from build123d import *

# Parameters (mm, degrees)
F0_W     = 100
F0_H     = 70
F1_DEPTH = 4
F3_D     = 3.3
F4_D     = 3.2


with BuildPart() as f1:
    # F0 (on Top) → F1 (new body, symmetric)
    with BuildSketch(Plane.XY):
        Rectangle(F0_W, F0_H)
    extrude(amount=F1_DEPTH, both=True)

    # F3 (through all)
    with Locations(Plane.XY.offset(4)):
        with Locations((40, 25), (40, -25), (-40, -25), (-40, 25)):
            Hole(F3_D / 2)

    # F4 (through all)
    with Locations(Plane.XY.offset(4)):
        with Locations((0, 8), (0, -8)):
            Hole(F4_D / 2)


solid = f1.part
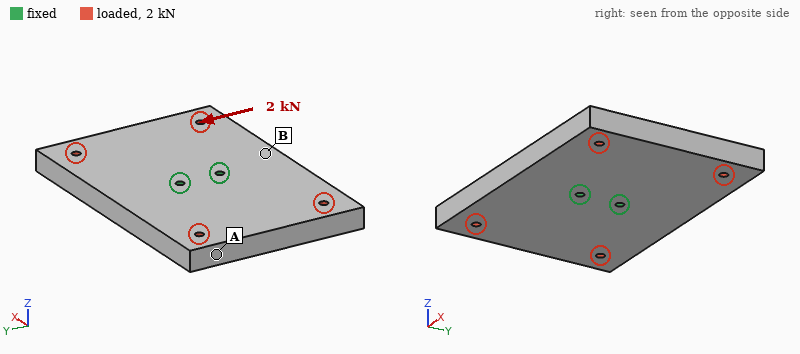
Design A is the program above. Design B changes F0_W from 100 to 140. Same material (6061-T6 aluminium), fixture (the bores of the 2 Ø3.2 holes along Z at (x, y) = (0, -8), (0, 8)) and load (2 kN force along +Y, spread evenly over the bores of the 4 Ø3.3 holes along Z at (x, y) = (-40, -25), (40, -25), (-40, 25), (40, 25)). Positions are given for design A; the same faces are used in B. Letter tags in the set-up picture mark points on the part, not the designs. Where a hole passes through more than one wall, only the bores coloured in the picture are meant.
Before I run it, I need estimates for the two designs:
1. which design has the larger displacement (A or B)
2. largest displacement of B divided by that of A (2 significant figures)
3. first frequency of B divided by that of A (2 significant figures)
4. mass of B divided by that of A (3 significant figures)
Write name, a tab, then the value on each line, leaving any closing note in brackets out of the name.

which design has the larger displacement	B
largest displacement of B divided by that of A	1.1
first frequency of B divided by that of A	0.56
mass of B divided by that of A	1.40
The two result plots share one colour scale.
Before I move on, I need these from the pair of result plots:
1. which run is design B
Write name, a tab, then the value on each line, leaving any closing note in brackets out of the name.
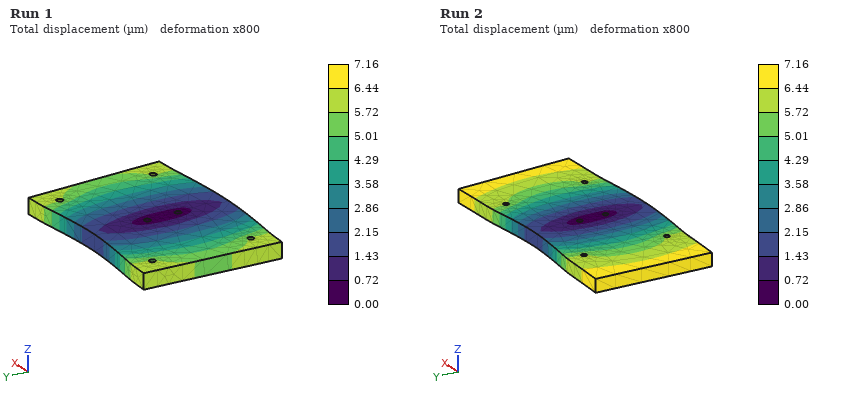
which run is design B	Run 2
